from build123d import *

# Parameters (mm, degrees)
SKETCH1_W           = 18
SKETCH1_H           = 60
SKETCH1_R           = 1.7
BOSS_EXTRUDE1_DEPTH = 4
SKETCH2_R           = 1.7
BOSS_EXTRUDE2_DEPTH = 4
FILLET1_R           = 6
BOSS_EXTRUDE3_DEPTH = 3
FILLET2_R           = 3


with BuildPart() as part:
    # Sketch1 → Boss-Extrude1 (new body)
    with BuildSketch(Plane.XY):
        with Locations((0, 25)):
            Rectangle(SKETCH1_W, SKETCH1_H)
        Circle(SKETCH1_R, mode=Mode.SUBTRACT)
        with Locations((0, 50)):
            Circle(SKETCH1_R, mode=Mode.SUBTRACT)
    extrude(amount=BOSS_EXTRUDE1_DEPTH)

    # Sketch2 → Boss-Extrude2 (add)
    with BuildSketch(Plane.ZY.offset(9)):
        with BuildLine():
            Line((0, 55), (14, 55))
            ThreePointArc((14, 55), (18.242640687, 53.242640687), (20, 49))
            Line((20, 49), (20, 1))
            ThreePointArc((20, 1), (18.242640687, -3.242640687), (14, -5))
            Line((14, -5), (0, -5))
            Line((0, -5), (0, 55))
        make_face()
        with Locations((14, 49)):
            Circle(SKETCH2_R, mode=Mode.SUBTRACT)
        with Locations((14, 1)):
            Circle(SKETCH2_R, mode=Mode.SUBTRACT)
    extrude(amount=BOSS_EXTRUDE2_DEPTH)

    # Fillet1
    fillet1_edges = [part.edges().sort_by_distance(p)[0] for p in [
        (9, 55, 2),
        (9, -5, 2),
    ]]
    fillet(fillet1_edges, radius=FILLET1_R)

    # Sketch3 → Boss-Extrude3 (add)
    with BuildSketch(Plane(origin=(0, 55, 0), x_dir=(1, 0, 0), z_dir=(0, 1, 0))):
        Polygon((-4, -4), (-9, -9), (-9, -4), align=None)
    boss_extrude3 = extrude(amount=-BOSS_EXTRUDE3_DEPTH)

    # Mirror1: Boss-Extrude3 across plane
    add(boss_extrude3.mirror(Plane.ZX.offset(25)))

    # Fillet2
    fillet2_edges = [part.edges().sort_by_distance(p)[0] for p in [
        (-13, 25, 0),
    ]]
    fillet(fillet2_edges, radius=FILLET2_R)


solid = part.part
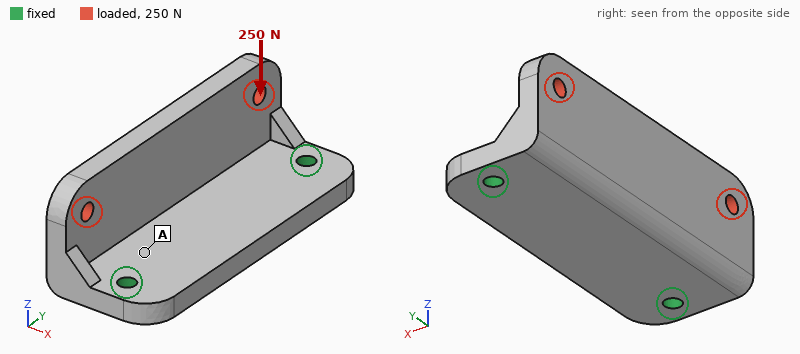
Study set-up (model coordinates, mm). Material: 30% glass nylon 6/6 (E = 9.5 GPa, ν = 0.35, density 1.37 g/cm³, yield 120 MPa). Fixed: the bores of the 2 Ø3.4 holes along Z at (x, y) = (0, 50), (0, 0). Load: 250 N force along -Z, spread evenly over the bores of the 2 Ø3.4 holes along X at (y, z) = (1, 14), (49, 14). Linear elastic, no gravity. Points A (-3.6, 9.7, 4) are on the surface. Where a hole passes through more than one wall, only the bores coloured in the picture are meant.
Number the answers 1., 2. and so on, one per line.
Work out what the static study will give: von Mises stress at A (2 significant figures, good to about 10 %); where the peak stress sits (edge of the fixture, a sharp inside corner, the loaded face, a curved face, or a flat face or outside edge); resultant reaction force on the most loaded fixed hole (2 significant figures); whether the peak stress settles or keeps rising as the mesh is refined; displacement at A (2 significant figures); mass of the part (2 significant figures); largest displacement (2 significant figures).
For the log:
1. 6.3 MPa
2. edge of the fixture
3. 130 N
4. keeps rising
5. 0.025 mm
6. 12 g
7. 0.17 mm
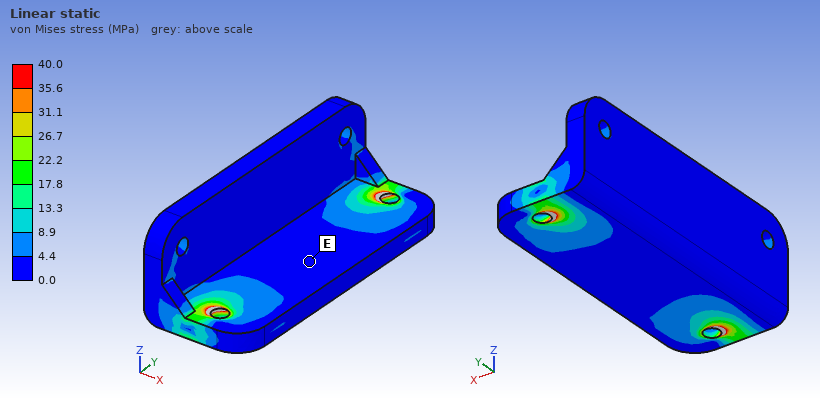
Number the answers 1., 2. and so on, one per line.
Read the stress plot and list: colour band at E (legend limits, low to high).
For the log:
1. 0.0 to 4.4 MPa
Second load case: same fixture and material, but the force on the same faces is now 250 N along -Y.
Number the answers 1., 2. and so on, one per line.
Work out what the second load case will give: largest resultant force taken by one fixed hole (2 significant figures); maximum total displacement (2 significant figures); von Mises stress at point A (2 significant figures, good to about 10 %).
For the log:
1. 150 N
2. 52 µm
3. 4.2 MPa
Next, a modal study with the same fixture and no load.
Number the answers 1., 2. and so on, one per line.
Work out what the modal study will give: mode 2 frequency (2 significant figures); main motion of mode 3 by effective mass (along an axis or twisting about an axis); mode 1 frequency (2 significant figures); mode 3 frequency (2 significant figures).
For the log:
1. 4000 Hz
2. along Z
3. 2200 Hz
4. 4800 Hz
